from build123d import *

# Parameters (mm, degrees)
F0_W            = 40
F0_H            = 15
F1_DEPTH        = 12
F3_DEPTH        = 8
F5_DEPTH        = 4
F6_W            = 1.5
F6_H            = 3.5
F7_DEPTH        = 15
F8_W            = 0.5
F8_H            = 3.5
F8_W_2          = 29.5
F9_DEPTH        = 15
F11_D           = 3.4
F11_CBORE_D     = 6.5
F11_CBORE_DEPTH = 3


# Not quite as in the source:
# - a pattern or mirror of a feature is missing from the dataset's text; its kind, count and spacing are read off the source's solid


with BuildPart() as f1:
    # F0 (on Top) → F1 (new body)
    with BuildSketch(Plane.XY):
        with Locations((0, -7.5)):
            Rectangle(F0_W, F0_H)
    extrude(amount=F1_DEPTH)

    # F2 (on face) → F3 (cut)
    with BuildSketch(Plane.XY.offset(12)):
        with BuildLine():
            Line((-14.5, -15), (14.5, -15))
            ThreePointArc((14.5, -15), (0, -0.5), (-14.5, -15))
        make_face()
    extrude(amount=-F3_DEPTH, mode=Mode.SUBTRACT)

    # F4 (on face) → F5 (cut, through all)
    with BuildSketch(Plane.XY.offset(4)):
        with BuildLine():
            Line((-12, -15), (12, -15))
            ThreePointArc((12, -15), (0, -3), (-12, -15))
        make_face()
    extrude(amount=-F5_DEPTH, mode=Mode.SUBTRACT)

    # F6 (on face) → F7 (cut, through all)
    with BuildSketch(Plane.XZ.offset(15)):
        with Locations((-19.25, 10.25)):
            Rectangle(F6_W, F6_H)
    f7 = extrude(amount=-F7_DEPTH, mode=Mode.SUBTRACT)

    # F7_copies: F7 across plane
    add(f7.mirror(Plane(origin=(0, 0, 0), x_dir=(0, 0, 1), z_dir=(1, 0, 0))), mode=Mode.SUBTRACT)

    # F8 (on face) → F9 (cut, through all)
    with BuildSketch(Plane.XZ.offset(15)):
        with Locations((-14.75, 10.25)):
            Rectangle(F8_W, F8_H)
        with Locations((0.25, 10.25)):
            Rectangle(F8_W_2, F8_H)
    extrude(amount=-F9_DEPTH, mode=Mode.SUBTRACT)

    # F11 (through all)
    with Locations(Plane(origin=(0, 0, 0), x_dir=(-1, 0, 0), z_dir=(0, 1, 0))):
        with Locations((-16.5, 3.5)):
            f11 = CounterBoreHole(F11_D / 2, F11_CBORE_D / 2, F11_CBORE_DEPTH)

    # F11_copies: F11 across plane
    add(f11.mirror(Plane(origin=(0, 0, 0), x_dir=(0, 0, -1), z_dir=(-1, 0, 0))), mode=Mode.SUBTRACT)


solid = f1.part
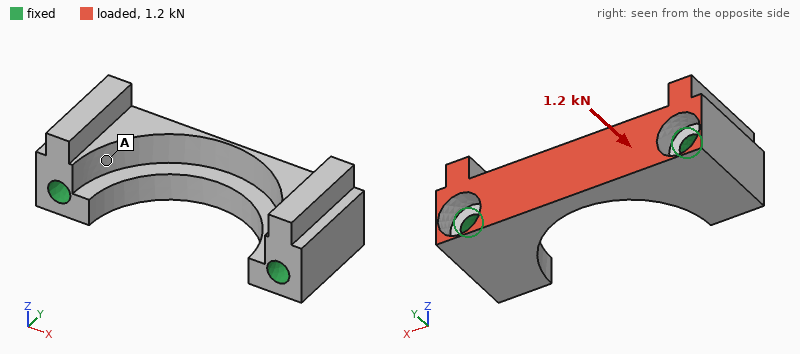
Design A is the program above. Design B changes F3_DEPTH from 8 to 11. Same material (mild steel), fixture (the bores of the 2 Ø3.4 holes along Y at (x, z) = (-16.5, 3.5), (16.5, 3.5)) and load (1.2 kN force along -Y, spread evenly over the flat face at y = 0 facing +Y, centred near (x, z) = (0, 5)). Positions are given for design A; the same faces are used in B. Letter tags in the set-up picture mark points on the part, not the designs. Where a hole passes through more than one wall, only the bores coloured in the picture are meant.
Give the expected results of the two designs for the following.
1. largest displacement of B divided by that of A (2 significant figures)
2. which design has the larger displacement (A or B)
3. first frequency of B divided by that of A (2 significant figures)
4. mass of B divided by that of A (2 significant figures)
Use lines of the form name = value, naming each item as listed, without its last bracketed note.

largest displacement of B divided by that of A = 1.3
which design has the larger displacement = B
first frequency of B divided by that of A = 1.1
mass of B divided by that of A = 0.88
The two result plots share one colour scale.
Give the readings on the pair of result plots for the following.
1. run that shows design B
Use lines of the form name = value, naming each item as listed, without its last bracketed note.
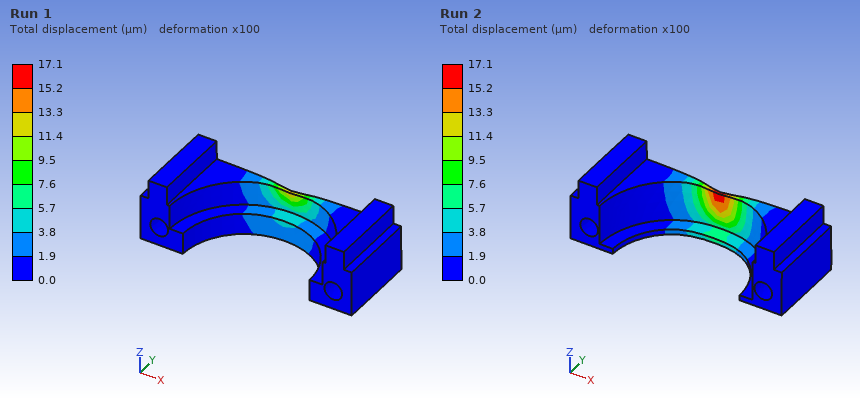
run that shows design B = Run 2
